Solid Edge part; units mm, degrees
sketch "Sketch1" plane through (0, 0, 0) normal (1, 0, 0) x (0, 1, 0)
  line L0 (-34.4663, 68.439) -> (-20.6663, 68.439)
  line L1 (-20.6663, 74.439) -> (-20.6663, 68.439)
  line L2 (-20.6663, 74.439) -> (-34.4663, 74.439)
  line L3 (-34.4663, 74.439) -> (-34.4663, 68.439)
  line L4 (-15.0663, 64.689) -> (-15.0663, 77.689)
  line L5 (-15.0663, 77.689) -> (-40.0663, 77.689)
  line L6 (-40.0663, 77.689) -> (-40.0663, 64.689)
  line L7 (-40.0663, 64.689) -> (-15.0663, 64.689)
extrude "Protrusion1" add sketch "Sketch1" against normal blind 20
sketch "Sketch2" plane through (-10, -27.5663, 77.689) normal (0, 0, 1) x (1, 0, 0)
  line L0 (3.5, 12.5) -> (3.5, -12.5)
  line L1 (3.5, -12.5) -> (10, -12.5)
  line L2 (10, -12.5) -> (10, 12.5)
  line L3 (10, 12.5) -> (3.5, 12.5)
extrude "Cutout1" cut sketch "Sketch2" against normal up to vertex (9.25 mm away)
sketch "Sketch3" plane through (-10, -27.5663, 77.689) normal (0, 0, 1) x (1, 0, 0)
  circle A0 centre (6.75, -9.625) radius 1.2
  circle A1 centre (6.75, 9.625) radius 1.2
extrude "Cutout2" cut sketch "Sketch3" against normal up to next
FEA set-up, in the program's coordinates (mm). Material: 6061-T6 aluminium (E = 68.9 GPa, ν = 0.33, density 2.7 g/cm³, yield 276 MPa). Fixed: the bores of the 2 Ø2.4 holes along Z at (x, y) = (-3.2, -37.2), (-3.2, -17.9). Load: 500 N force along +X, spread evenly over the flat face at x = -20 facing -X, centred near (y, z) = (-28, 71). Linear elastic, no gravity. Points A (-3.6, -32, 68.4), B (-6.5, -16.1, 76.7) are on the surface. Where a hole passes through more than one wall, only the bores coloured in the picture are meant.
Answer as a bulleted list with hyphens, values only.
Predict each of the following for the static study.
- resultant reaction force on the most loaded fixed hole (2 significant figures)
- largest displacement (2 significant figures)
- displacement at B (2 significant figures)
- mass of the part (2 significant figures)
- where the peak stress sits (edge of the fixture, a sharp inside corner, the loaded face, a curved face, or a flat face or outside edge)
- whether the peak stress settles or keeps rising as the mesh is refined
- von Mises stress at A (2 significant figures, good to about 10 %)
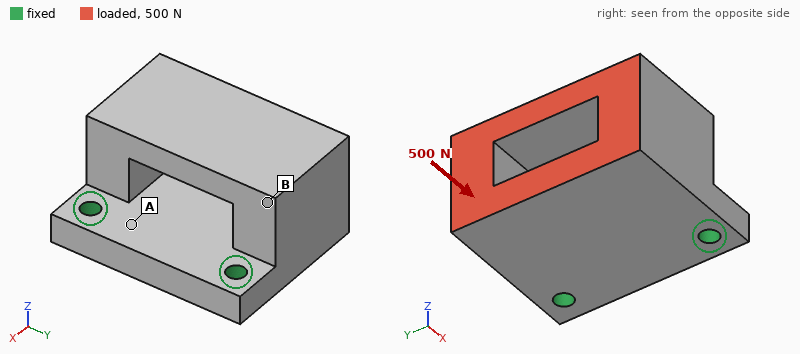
- 250 N
- 40 µm
- 23 µm
- 10 g
- edge of the fixture
- keeps rising
- 18 MPa
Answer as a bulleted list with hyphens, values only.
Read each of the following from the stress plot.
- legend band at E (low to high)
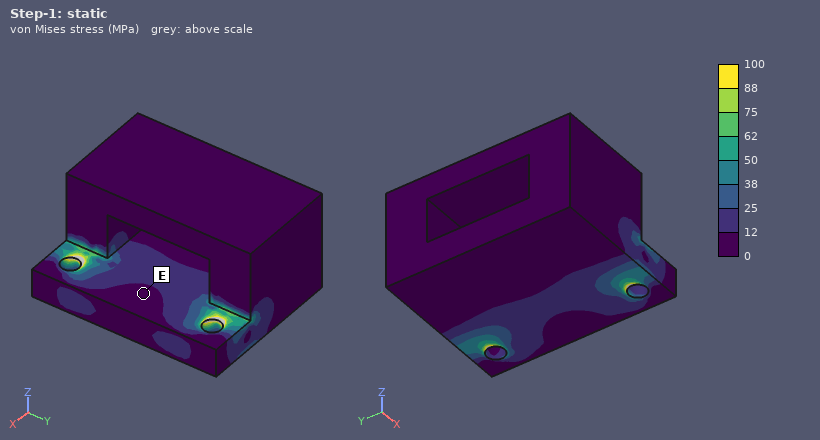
- 0 to 12 MPa
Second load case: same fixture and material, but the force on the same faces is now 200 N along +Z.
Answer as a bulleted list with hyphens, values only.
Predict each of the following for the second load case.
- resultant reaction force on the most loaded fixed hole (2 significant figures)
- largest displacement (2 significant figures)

- 100 N
- 52 µm
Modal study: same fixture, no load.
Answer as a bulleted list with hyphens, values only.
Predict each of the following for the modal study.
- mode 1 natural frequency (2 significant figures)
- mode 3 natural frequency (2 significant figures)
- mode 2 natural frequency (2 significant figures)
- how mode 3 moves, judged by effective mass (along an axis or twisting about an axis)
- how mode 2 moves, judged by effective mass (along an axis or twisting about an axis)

- 5100 Hz
- 19 kHz
- 13 kHz
- along Y
- along Y
